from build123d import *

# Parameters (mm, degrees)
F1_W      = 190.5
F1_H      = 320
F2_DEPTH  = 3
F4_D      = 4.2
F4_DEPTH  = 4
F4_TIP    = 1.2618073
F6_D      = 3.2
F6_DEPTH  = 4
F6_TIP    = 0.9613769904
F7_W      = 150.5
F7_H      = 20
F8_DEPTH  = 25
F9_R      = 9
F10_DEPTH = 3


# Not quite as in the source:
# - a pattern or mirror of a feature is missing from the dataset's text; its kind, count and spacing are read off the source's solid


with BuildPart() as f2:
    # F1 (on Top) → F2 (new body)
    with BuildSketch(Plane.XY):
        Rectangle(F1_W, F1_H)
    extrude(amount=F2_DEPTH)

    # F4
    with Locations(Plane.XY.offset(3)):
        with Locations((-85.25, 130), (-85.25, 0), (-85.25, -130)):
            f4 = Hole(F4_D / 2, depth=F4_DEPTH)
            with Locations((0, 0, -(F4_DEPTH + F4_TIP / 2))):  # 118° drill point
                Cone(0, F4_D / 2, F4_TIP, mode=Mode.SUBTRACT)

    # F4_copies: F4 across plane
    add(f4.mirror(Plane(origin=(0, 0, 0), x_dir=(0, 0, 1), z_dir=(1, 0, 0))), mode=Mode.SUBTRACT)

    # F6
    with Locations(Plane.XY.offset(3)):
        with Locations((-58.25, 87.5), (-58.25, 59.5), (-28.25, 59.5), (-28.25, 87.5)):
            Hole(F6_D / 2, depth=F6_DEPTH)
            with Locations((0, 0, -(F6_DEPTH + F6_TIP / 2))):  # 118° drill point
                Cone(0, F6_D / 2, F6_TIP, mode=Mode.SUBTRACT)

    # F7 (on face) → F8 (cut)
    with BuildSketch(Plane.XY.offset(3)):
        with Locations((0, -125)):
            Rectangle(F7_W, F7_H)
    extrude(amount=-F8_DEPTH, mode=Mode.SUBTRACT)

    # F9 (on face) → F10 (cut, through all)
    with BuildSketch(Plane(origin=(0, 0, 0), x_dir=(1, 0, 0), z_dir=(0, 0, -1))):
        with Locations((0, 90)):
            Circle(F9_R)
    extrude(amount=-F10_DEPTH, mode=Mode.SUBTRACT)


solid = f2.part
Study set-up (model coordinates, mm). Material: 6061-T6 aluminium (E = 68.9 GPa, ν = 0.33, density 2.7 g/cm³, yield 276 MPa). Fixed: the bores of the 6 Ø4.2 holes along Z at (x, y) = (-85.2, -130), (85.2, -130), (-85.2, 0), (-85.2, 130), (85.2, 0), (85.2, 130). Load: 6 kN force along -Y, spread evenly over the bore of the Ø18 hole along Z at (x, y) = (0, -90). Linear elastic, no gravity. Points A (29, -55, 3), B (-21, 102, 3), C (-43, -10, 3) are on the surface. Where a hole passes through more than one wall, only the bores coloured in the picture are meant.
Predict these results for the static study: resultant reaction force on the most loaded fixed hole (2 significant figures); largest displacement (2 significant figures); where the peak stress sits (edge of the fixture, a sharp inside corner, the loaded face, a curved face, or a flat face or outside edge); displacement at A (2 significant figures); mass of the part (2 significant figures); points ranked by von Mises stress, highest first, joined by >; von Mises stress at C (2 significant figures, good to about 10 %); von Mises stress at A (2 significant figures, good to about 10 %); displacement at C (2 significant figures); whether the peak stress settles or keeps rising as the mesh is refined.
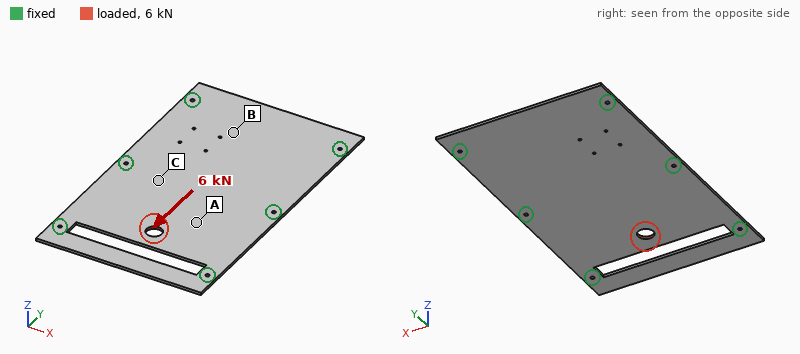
1.7 kN
51 µm
edge of the fixture
22 µm
470 g
A > C > B
10 MPa
19 MPa
13 µm
keeps rising
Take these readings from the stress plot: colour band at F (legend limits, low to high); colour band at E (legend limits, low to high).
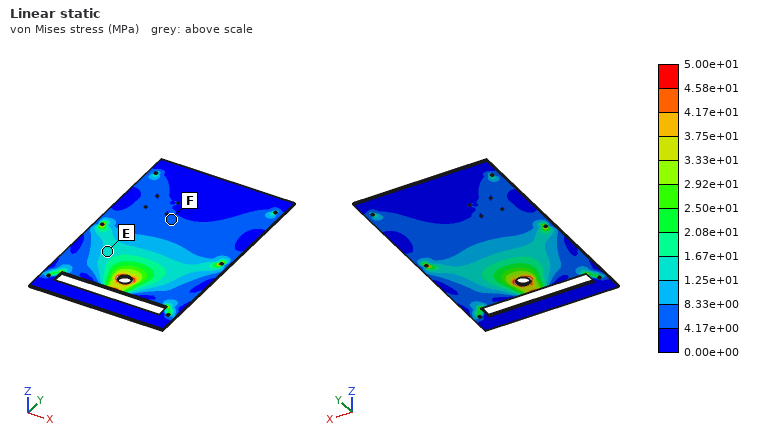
4.17e+00 to 8.33e+00 MPa
1.25e+01 to 1.67e+01 MPa
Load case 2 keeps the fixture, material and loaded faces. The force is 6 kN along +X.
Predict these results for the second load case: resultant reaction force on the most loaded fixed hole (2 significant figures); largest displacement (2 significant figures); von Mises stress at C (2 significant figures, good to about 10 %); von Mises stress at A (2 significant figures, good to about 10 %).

2.4 kN
55 µm
11 MPa
15 MPa
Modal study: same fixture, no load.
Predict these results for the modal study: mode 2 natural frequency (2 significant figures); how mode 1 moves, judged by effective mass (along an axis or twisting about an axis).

440 Hz
along Z
